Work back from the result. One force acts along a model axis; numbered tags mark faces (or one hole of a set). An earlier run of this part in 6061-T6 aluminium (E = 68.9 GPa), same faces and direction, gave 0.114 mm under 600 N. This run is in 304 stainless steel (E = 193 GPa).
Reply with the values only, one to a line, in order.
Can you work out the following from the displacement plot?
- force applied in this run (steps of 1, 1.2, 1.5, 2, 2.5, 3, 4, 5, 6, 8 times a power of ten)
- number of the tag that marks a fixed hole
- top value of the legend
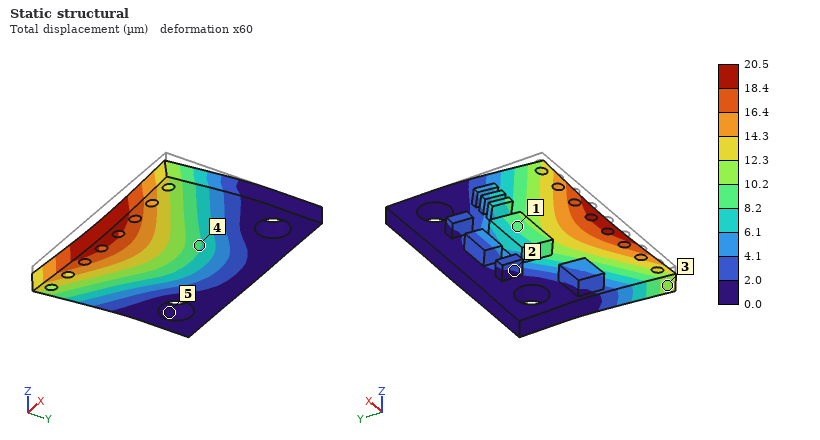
300 N
5
20.5 µm
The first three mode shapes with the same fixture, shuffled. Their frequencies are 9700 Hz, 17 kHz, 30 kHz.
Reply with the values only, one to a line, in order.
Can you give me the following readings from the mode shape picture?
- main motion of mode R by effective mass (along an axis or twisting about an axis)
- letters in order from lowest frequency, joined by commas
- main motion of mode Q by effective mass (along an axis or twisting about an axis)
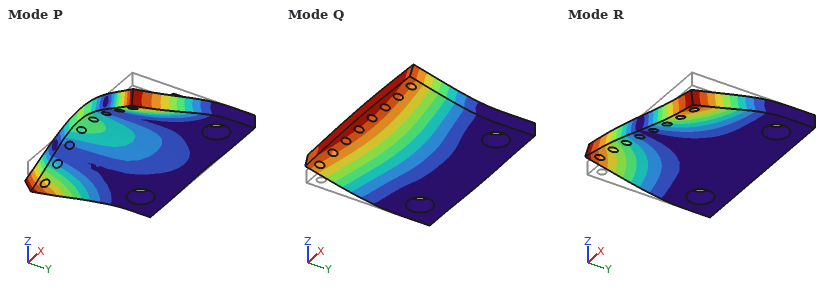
twisting about Y
Q, R, P
along Z
